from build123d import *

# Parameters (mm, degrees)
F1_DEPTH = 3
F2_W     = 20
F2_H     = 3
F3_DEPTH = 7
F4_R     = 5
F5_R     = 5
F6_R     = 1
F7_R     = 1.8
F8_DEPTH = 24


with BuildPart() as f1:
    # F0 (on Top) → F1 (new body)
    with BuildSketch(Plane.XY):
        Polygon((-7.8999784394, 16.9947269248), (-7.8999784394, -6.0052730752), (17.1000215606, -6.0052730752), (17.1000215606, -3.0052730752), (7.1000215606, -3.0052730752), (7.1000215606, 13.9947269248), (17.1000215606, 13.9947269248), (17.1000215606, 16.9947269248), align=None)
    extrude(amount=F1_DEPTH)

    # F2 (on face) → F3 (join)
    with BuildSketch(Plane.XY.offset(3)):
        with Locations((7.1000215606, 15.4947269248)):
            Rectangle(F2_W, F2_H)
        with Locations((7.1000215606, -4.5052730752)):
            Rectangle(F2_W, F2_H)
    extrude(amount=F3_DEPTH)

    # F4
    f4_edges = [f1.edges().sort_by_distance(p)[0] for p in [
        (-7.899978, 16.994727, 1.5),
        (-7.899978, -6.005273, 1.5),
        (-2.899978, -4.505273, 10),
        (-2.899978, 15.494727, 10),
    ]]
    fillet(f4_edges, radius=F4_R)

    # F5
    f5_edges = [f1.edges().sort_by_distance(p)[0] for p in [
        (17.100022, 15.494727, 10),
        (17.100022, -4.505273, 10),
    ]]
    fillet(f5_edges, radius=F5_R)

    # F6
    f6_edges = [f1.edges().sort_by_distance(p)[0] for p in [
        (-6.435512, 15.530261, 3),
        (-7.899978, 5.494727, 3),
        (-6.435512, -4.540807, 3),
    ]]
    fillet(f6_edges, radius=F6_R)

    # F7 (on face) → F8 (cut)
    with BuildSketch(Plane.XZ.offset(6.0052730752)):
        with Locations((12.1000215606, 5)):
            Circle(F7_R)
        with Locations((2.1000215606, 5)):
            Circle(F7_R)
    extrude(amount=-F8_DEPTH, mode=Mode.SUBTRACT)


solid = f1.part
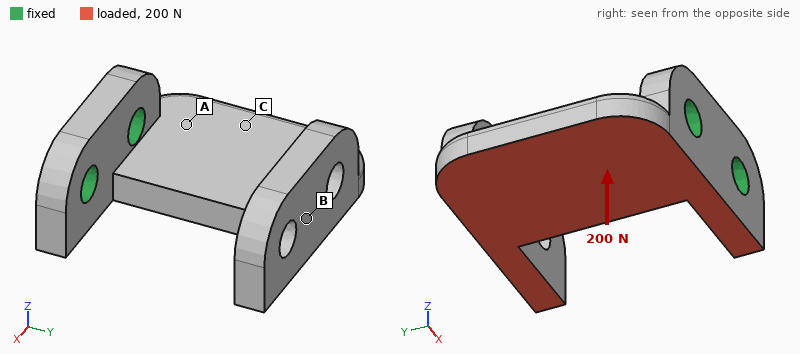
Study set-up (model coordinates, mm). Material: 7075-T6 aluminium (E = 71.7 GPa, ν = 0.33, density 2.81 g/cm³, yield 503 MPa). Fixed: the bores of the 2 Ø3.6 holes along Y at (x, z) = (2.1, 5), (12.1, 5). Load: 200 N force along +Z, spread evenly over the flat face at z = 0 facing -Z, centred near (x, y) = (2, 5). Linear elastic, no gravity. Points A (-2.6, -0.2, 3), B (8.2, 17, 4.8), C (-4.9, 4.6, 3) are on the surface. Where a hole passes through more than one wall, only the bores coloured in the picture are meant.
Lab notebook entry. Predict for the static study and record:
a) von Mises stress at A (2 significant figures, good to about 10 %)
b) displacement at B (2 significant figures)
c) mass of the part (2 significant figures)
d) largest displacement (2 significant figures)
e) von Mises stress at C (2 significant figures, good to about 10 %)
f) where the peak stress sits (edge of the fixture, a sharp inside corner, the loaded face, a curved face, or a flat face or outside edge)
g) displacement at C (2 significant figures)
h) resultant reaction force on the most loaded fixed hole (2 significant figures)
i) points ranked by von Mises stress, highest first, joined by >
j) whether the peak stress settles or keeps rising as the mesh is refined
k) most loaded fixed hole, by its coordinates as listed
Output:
50 MPa
0.15 mm
5.1 g
0.16 mm
28 MPa
edge of the fixture
0.049 mm
200 N
A > C > B
keeps rising
(2.1, 5)
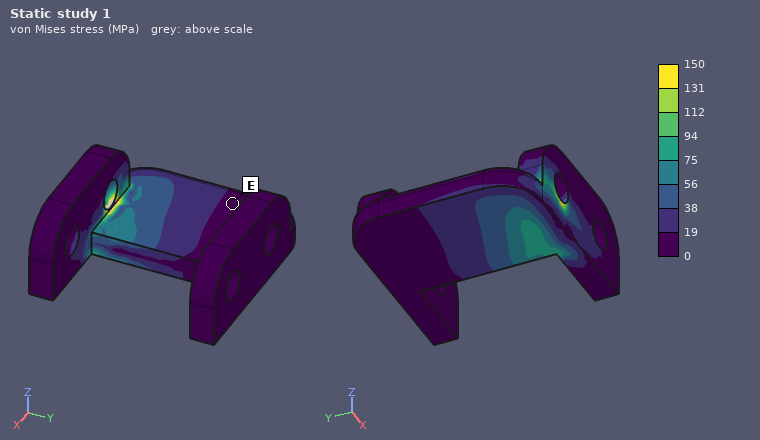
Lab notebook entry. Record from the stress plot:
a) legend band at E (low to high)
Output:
0 to 19 MPa
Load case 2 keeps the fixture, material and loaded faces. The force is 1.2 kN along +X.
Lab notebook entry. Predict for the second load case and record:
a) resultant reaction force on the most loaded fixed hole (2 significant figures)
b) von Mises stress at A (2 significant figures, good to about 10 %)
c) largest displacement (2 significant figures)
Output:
1.0 kN
71 MPa
0.22 mm
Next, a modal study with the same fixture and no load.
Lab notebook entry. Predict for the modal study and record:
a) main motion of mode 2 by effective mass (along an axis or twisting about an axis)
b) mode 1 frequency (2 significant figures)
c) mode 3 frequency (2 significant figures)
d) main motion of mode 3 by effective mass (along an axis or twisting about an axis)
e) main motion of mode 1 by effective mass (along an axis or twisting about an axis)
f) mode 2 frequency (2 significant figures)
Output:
along X
2700 Hz
7500 Hz
along X
along Z
5000 Hz
